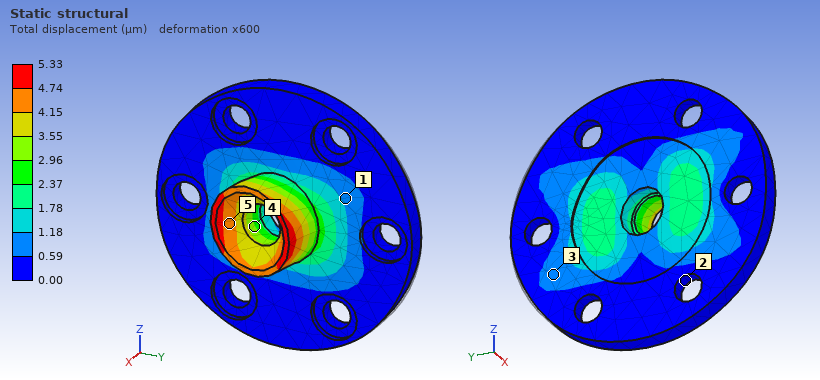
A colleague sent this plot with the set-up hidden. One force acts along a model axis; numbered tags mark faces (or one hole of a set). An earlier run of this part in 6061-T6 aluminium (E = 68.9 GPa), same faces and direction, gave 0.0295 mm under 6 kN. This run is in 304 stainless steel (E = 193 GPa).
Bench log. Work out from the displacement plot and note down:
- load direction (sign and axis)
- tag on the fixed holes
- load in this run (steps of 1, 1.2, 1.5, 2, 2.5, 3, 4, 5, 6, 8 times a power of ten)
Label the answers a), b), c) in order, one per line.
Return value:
a) -Y
b) 2
c) 3 kN
